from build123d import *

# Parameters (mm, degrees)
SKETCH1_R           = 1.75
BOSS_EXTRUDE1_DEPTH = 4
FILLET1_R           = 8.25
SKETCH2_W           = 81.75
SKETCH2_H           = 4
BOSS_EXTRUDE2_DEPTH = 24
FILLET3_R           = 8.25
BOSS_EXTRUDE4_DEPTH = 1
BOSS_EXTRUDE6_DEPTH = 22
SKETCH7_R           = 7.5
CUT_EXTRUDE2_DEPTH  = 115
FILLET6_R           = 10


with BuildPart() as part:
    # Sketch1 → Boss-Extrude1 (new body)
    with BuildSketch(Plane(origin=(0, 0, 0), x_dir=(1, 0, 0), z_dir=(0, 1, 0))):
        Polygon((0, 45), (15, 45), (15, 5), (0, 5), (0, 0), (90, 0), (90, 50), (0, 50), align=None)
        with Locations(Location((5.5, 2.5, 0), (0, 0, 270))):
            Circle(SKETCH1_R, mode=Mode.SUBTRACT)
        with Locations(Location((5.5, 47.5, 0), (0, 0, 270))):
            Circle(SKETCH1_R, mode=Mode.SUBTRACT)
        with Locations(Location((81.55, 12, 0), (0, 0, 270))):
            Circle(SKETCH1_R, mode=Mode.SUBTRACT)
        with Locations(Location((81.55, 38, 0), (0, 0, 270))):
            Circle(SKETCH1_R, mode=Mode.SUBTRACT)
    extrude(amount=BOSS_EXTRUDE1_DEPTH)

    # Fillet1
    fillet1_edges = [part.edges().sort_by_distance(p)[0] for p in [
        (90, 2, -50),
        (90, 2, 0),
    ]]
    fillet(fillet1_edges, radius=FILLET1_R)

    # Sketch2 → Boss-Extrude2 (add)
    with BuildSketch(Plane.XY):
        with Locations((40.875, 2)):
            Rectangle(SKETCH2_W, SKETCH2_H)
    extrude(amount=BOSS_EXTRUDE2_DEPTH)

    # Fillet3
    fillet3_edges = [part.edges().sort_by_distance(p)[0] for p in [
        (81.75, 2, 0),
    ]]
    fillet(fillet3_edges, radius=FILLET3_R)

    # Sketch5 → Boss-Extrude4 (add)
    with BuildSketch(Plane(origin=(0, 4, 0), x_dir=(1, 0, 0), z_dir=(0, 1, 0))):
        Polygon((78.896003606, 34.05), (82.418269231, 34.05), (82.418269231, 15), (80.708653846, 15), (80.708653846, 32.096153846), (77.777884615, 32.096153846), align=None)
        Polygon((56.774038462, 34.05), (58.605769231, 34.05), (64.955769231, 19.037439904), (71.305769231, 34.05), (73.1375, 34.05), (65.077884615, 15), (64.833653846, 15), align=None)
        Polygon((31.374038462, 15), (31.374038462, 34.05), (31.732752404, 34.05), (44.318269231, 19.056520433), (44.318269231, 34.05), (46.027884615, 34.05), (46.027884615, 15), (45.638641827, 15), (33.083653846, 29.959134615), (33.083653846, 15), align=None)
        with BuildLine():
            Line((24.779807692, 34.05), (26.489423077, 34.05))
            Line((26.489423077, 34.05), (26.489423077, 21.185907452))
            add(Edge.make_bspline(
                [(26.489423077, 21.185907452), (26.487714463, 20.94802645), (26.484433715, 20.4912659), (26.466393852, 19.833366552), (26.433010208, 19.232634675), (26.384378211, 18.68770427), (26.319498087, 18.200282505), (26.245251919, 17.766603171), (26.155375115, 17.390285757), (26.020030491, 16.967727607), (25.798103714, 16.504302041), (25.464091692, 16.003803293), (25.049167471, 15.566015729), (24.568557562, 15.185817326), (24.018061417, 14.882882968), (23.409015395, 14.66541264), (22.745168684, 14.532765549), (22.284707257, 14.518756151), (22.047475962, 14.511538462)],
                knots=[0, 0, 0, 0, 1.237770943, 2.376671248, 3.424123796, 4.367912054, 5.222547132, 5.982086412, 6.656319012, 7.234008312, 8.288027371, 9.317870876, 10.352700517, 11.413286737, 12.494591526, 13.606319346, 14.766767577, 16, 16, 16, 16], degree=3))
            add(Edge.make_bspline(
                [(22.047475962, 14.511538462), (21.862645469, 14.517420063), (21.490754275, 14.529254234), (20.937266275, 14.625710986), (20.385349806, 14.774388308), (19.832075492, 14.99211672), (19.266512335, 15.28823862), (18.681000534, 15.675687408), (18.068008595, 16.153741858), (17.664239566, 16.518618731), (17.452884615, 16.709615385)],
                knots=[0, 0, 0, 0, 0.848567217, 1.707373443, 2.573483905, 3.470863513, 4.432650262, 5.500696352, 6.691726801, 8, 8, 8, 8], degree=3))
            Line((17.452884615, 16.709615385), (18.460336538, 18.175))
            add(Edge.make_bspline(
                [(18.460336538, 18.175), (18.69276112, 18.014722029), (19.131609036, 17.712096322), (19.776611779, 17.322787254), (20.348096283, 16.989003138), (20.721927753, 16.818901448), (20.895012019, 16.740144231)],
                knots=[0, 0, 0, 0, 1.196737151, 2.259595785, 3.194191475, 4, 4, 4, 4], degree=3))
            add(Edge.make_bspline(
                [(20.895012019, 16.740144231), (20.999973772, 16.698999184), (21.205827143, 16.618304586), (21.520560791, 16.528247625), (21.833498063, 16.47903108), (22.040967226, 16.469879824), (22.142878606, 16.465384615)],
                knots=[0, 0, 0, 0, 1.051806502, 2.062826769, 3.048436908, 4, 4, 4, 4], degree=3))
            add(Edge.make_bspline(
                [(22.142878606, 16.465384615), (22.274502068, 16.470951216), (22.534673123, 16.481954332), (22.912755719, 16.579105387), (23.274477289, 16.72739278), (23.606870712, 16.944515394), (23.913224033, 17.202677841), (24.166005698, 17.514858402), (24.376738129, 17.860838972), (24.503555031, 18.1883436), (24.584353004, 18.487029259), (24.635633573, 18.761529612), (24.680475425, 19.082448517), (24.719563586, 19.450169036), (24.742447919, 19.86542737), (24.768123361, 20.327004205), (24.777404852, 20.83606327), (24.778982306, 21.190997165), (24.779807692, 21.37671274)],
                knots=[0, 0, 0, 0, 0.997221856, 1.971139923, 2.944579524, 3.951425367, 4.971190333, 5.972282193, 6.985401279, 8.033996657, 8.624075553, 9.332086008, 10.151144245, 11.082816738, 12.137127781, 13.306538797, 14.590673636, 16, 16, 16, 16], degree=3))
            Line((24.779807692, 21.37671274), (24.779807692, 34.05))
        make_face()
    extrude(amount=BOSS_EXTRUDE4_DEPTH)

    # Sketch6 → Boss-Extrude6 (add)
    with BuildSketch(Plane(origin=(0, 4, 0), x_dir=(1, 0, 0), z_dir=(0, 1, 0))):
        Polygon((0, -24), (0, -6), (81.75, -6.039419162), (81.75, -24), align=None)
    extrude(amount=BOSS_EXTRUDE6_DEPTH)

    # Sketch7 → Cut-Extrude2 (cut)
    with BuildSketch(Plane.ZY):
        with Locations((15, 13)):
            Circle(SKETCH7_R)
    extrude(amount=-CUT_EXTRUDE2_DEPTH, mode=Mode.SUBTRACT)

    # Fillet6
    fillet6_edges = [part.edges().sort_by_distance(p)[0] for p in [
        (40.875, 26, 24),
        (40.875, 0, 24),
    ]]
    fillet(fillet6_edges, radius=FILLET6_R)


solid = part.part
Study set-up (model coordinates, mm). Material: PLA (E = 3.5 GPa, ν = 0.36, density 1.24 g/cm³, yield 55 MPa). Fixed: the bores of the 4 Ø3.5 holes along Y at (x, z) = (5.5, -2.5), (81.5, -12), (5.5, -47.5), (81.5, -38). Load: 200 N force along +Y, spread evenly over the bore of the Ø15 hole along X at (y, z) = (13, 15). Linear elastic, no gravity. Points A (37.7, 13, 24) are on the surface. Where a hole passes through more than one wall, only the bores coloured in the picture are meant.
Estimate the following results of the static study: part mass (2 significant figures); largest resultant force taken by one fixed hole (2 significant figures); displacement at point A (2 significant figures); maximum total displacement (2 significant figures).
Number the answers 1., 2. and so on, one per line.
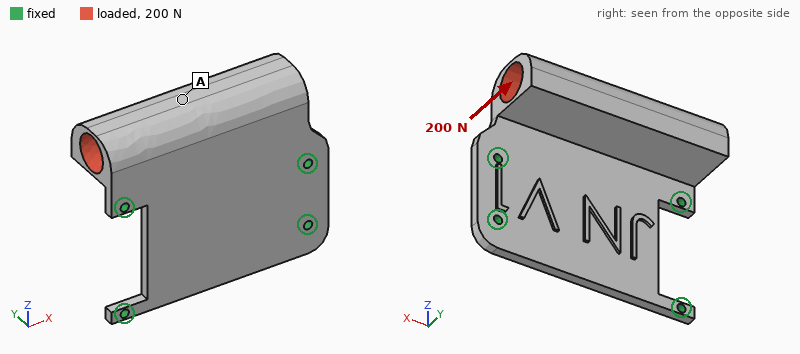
1. 47 g
2. 130 N
3. 1.1 mm
4. 1.4 mm
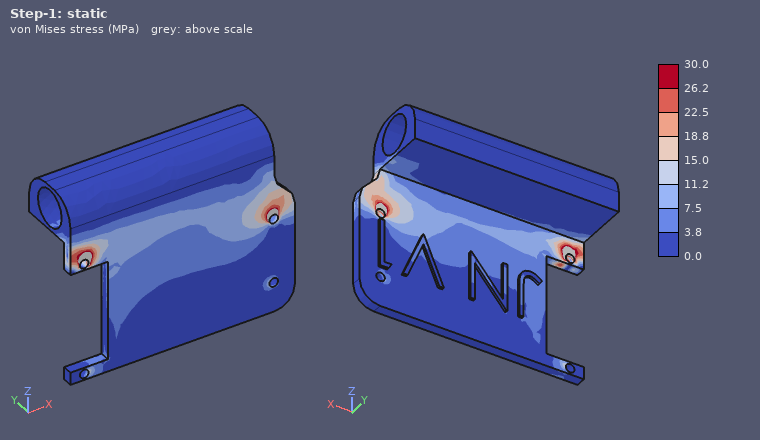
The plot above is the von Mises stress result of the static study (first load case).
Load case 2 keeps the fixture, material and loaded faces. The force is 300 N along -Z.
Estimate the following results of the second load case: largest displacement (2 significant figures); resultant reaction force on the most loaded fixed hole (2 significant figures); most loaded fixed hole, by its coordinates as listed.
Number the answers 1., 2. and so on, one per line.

1. 1.3 mm
2. 130 N
3. (5.5, -2.5)
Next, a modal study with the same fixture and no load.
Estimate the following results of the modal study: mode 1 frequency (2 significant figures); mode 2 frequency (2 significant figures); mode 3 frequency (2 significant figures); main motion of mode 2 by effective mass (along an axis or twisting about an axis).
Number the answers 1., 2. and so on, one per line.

1. 420 Hz
2. 1100 Hz
3. 1300 Hz
4. along Y
